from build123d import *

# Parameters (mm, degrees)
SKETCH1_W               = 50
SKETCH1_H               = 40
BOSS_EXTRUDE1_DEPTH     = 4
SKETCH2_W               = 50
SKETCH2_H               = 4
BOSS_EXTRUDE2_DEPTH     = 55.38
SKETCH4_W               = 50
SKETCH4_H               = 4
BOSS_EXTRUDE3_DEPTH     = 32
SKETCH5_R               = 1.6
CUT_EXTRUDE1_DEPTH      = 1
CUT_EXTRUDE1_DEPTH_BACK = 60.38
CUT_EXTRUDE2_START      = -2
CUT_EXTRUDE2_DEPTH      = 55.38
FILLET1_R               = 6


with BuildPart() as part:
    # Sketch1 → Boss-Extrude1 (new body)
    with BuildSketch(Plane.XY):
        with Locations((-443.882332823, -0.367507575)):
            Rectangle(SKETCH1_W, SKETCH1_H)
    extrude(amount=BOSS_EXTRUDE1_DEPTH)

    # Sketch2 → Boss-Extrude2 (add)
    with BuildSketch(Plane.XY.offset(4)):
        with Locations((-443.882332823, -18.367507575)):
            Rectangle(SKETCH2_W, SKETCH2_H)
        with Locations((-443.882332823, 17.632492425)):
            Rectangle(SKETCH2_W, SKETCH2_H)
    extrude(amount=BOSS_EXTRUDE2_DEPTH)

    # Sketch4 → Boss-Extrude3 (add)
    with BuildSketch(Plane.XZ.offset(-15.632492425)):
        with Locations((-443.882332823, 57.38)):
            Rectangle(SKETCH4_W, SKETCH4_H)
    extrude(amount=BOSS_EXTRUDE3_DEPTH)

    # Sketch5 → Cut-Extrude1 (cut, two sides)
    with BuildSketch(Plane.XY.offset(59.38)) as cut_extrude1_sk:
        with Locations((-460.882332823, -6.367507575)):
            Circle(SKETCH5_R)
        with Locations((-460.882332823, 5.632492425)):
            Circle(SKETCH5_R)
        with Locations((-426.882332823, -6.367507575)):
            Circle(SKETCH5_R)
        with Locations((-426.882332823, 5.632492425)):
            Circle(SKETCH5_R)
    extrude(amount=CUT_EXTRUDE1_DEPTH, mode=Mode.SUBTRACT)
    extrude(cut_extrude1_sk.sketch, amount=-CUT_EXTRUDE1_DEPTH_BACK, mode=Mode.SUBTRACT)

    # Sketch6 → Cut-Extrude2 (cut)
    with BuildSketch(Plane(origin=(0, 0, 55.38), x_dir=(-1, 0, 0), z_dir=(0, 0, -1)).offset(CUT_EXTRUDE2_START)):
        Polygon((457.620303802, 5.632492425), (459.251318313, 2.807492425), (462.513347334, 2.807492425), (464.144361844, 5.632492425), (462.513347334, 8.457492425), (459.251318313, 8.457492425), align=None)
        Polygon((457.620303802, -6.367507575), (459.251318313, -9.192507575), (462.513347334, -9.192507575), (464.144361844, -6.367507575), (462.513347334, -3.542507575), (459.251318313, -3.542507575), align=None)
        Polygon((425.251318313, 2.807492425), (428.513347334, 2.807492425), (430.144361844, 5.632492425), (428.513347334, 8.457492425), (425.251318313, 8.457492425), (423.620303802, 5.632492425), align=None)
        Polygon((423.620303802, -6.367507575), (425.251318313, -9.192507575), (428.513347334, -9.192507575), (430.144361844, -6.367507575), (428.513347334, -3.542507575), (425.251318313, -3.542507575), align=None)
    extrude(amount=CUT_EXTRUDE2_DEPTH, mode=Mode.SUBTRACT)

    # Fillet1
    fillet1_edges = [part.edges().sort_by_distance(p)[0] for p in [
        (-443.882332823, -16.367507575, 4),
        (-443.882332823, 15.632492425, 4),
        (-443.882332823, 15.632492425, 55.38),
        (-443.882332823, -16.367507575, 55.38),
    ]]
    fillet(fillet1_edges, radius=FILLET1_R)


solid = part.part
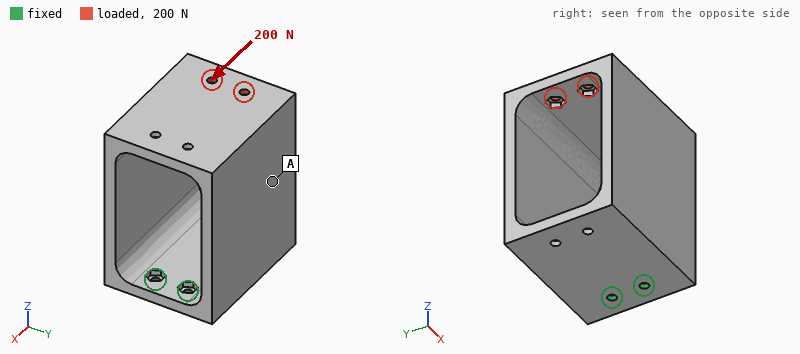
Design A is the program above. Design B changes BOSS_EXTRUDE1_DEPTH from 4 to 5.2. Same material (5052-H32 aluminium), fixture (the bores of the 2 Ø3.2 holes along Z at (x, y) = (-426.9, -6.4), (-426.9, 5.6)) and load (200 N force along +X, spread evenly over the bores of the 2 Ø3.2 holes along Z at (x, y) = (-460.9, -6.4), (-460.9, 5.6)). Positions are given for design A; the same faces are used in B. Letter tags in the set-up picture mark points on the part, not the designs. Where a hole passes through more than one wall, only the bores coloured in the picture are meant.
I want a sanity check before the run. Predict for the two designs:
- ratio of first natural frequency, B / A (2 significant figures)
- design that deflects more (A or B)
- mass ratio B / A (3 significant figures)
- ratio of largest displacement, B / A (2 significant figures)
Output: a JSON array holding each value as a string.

["1.1", "A", "1.05", "0.83"]
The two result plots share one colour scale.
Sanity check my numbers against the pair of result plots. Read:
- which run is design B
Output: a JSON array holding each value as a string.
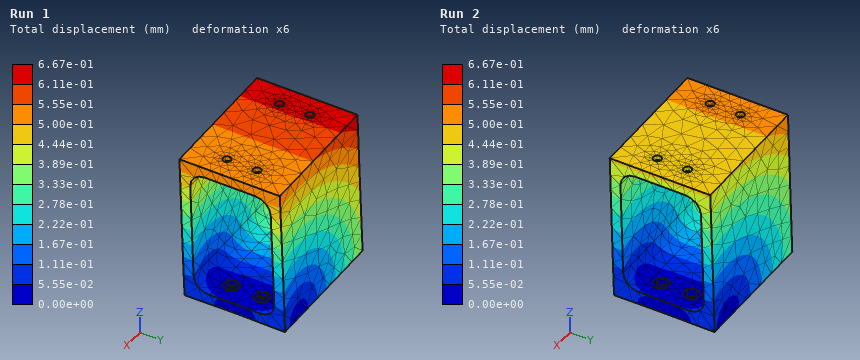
["Run 2"]
